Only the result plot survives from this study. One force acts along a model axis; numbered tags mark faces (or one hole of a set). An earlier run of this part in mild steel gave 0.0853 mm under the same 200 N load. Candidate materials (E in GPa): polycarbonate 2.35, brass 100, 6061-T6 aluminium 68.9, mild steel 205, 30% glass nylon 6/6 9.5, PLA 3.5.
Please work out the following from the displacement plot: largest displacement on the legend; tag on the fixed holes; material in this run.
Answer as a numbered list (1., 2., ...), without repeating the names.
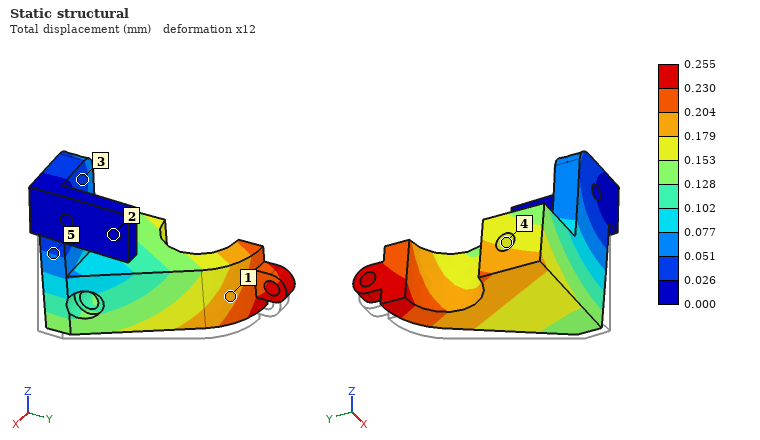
1. 0.255 mm
2. 2
3. 6061-T6 aluminium
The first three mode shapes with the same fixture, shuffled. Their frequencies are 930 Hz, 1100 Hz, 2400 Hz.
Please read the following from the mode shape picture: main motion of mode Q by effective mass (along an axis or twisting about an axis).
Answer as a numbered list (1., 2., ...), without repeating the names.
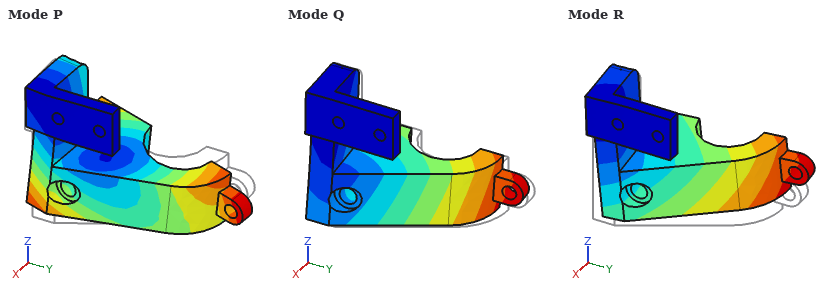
1. along Y
